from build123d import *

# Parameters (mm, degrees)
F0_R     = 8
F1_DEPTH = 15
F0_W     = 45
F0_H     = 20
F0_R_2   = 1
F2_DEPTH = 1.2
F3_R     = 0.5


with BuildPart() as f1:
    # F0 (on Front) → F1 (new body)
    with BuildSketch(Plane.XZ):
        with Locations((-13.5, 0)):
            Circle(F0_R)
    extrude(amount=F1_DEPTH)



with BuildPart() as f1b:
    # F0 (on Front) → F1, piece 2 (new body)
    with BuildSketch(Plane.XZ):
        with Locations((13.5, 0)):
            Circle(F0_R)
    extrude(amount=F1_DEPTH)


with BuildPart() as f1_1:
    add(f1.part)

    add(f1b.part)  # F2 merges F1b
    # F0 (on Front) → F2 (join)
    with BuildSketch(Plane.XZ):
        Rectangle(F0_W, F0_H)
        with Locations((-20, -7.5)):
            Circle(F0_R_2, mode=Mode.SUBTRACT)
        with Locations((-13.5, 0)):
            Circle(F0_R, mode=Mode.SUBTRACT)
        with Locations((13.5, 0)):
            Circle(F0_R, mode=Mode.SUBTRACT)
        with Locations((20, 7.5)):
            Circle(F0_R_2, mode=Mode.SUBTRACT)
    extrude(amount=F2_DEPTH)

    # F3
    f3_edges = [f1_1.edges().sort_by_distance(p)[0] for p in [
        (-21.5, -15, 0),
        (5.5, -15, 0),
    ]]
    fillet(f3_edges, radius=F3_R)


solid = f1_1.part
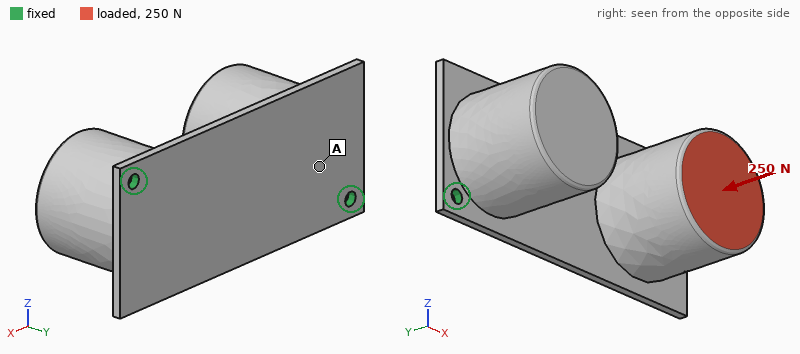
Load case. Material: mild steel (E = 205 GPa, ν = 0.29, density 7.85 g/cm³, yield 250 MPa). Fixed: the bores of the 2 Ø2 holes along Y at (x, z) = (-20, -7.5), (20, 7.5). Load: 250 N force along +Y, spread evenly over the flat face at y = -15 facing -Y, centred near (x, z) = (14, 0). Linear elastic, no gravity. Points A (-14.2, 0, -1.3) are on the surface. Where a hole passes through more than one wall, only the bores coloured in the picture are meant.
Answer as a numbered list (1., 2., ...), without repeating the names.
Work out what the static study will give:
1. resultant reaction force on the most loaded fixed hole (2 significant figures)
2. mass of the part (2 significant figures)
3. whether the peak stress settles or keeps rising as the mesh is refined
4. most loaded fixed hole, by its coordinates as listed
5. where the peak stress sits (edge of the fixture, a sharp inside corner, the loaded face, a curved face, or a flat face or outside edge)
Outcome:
1. 200 N
2. 52 g
3. keeps rising
4. (20, 7.5)
5. edge of the fixture
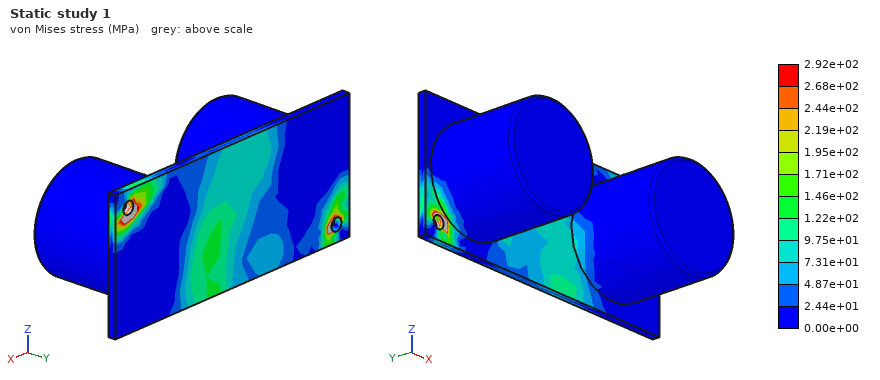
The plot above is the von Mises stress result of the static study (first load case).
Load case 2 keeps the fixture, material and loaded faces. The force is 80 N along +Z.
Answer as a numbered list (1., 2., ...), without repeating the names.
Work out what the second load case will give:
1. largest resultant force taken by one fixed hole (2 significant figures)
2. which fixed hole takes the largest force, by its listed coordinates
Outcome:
1. 74 N
2. (20, 7.5)
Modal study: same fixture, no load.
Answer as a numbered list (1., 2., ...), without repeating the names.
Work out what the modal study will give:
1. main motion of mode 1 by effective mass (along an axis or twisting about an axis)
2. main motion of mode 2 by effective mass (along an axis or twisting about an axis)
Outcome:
1. along Y
2. along Z
